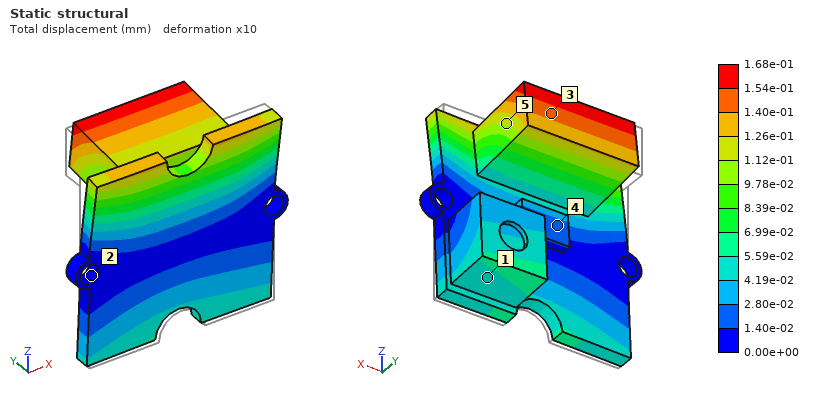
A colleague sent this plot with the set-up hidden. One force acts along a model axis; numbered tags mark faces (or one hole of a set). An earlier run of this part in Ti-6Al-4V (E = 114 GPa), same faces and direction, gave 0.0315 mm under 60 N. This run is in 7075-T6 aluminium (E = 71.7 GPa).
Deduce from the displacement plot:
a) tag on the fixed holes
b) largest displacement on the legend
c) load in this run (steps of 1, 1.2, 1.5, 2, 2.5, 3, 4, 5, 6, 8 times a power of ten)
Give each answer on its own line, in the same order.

2
1.68e-01 mm
200 N
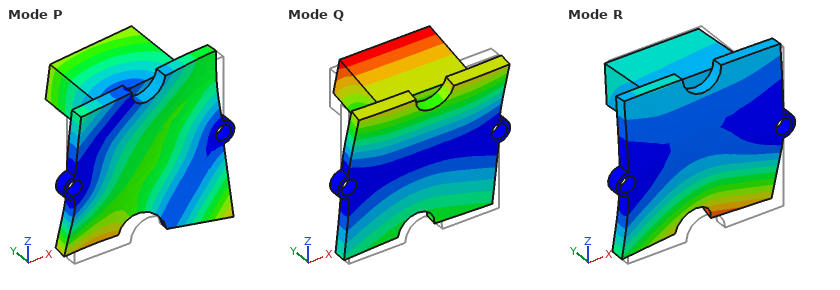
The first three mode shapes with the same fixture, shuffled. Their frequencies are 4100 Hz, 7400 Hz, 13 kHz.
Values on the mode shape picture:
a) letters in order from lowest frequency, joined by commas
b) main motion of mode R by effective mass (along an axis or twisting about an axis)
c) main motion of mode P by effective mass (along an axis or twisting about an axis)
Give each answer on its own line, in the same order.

Q, R, P
along Y
along Y
